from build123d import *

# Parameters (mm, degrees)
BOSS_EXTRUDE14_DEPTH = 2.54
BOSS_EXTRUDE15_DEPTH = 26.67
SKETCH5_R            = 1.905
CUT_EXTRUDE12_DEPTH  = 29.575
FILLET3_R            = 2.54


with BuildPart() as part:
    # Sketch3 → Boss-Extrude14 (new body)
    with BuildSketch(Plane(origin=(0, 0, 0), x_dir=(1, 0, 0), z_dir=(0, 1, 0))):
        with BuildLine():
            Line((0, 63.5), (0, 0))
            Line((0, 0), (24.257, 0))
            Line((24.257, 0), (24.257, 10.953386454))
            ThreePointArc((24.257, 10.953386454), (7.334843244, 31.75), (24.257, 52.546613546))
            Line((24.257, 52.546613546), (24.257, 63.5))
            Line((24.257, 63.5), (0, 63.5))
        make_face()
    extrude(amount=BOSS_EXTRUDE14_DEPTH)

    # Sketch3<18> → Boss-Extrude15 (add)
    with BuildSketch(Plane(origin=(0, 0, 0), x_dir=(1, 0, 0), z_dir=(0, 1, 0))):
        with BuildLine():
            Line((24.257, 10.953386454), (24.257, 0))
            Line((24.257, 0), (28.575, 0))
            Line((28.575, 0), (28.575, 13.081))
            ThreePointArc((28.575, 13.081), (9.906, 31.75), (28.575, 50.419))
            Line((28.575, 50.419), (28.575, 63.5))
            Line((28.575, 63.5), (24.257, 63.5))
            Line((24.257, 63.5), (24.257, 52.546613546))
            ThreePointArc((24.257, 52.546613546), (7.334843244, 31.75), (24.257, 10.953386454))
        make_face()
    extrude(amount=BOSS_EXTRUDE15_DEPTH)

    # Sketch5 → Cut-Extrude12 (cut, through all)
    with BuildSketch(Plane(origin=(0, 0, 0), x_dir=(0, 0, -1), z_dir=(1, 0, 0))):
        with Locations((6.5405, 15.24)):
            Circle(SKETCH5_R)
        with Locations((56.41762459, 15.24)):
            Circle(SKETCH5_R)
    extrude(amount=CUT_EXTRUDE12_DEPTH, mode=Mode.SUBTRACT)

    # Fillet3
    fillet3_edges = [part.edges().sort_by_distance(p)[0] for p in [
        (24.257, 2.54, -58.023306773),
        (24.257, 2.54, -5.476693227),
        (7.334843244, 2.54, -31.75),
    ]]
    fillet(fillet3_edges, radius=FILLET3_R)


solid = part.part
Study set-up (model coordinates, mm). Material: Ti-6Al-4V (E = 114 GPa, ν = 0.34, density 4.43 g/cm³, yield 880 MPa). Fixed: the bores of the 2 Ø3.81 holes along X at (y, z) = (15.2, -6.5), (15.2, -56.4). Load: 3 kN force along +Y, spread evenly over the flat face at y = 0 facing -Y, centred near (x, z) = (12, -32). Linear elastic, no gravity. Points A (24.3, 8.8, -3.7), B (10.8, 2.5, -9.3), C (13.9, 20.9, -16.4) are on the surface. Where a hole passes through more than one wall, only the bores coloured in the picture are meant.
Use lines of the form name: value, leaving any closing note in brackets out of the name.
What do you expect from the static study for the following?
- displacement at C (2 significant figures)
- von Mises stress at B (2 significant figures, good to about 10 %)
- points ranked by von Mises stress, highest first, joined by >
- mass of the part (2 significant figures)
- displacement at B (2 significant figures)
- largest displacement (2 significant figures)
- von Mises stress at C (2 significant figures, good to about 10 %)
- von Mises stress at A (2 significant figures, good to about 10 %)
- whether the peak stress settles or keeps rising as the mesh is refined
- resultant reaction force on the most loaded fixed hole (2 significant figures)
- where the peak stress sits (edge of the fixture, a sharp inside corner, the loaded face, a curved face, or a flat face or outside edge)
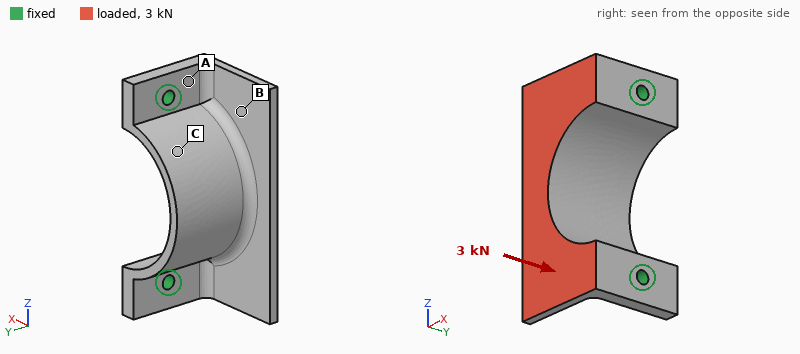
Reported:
displacement at C: 0.084 mm
von Mises stress at B: 87 MPa
points ranked by von Mises stress, highest first, joined by >: A > B > C
mass of the part: 41 g
displacement at B: 0.17 mm
largest displacement: 0.39 mm
von Mises stress at C: 47 MPa
von Mises stress at A: 150 MPa
whether the peak stress settles or keeps rising as the mesh is refined: keeps rising
resultant reaction force on the most loaded fixed hole: 1.5 kN
where the peak stress sits: edge of the fixture
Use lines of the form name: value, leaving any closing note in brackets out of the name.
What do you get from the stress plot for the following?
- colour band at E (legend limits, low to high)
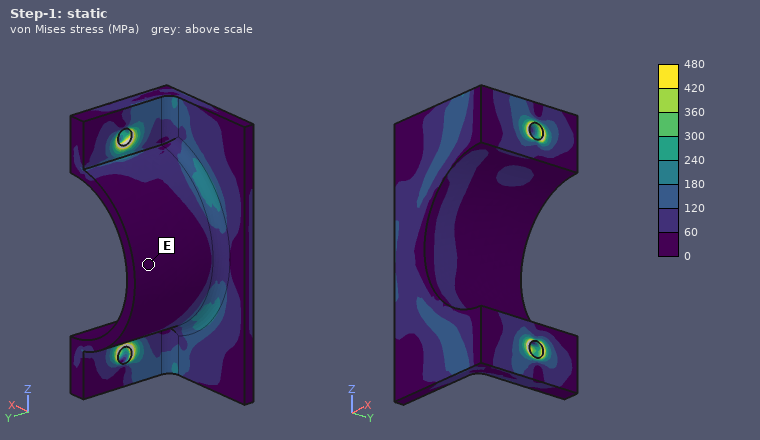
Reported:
colour band at E: 0 to 60 MPa
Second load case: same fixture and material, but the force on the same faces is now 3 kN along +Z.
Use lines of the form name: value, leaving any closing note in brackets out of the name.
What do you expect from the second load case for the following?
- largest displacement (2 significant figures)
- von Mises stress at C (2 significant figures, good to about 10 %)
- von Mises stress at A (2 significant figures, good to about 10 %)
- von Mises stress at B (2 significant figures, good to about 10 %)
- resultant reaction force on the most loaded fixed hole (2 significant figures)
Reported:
largest displacement: 61 µm
von Mises stress at C: 26 MPa
von Mises stress at A: 60 MPa
von Mises stress at B: 29 MPa
resultant reaction force on the most loaded fixed hole: 1.9 kN
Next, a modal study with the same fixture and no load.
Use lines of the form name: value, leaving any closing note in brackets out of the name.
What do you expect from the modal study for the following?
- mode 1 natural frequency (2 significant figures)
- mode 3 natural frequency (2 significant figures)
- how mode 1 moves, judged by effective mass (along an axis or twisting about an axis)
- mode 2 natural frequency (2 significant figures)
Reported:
mode 1 natural frequency: 4000 Hz
mode 3 natural frequency: 8000 Hz
how mode 1 moves, judged by effective mass: along Y
mode 2 natural frequency: 5600 Hz
